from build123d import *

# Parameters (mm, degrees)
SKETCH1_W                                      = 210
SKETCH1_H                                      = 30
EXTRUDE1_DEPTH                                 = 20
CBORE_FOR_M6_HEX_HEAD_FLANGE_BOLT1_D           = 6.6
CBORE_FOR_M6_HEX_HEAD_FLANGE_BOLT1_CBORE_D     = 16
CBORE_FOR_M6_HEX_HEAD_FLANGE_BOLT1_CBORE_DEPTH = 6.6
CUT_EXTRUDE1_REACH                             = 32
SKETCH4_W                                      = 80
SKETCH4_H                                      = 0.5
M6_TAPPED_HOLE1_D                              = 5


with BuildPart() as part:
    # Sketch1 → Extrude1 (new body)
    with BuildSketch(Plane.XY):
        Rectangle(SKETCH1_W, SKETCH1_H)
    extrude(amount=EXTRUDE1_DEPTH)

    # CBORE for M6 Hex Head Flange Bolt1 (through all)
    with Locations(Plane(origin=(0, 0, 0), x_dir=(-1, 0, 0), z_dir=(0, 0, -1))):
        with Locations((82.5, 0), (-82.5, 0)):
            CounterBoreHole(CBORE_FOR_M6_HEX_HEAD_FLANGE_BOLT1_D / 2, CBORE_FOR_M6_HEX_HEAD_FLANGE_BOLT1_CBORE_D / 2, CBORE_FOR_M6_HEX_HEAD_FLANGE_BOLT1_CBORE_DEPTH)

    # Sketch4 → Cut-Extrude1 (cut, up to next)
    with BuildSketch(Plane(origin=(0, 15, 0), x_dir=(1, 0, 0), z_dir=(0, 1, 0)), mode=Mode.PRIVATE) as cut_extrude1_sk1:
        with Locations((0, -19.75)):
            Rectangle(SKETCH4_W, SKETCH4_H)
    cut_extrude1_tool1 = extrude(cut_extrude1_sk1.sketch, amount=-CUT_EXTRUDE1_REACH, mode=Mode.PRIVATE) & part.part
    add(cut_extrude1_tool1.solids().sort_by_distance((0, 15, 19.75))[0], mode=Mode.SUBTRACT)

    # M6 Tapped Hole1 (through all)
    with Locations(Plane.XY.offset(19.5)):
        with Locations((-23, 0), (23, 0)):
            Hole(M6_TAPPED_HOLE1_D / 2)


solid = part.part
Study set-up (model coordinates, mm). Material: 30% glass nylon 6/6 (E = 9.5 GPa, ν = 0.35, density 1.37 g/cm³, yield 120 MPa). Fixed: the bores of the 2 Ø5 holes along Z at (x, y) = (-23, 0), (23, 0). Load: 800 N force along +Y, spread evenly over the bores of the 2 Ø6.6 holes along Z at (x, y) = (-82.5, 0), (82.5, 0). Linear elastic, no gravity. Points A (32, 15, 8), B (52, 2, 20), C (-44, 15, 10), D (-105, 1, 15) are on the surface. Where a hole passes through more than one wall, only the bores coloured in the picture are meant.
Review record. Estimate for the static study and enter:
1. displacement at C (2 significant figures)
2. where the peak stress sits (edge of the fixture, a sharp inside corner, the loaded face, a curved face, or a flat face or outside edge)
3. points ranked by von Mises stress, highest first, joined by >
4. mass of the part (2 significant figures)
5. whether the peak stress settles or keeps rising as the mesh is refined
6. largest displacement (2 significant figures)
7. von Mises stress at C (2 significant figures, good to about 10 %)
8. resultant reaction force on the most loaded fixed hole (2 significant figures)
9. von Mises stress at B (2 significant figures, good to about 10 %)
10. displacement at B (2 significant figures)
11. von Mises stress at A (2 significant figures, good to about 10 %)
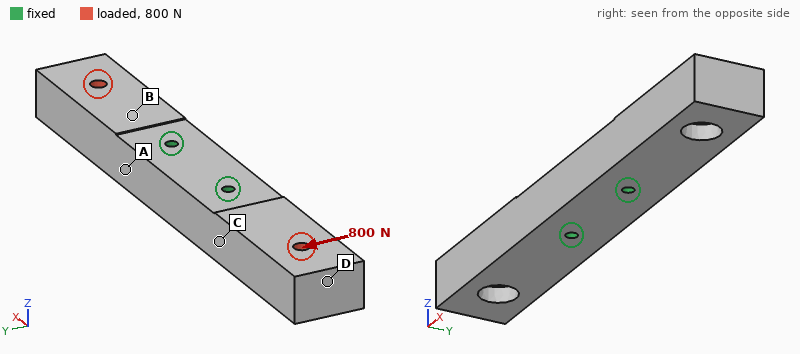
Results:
0.048 mm
edge of the fixture
A > C > B > D
170 g
keeps rising
0.21 mm
5.3 MPa
400 N
2.6 MPa
0.057 mm
7.0 MPa
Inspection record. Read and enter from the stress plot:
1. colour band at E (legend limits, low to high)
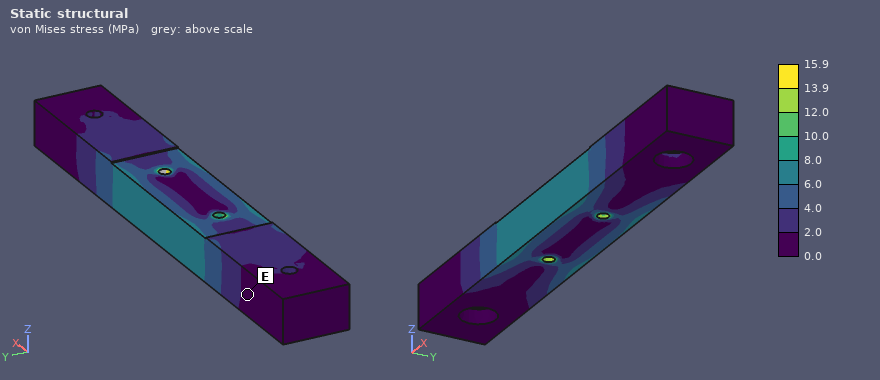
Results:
0.0 to 2.0 MPa
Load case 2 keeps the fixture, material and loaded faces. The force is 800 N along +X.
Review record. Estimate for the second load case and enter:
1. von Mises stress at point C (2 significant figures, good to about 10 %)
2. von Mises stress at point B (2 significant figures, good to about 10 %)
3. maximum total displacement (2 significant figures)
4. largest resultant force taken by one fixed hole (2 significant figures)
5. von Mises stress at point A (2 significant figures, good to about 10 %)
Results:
0.62 MPa
1.4 MPa
26 µm
400 N
0.31 MPa
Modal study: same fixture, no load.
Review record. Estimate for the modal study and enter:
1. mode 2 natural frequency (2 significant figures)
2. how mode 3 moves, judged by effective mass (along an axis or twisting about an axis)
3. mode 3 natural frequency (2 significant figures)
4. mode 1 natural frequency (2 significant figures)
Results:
1100 Hz
along Y
1300 Hz
1100 Hz
